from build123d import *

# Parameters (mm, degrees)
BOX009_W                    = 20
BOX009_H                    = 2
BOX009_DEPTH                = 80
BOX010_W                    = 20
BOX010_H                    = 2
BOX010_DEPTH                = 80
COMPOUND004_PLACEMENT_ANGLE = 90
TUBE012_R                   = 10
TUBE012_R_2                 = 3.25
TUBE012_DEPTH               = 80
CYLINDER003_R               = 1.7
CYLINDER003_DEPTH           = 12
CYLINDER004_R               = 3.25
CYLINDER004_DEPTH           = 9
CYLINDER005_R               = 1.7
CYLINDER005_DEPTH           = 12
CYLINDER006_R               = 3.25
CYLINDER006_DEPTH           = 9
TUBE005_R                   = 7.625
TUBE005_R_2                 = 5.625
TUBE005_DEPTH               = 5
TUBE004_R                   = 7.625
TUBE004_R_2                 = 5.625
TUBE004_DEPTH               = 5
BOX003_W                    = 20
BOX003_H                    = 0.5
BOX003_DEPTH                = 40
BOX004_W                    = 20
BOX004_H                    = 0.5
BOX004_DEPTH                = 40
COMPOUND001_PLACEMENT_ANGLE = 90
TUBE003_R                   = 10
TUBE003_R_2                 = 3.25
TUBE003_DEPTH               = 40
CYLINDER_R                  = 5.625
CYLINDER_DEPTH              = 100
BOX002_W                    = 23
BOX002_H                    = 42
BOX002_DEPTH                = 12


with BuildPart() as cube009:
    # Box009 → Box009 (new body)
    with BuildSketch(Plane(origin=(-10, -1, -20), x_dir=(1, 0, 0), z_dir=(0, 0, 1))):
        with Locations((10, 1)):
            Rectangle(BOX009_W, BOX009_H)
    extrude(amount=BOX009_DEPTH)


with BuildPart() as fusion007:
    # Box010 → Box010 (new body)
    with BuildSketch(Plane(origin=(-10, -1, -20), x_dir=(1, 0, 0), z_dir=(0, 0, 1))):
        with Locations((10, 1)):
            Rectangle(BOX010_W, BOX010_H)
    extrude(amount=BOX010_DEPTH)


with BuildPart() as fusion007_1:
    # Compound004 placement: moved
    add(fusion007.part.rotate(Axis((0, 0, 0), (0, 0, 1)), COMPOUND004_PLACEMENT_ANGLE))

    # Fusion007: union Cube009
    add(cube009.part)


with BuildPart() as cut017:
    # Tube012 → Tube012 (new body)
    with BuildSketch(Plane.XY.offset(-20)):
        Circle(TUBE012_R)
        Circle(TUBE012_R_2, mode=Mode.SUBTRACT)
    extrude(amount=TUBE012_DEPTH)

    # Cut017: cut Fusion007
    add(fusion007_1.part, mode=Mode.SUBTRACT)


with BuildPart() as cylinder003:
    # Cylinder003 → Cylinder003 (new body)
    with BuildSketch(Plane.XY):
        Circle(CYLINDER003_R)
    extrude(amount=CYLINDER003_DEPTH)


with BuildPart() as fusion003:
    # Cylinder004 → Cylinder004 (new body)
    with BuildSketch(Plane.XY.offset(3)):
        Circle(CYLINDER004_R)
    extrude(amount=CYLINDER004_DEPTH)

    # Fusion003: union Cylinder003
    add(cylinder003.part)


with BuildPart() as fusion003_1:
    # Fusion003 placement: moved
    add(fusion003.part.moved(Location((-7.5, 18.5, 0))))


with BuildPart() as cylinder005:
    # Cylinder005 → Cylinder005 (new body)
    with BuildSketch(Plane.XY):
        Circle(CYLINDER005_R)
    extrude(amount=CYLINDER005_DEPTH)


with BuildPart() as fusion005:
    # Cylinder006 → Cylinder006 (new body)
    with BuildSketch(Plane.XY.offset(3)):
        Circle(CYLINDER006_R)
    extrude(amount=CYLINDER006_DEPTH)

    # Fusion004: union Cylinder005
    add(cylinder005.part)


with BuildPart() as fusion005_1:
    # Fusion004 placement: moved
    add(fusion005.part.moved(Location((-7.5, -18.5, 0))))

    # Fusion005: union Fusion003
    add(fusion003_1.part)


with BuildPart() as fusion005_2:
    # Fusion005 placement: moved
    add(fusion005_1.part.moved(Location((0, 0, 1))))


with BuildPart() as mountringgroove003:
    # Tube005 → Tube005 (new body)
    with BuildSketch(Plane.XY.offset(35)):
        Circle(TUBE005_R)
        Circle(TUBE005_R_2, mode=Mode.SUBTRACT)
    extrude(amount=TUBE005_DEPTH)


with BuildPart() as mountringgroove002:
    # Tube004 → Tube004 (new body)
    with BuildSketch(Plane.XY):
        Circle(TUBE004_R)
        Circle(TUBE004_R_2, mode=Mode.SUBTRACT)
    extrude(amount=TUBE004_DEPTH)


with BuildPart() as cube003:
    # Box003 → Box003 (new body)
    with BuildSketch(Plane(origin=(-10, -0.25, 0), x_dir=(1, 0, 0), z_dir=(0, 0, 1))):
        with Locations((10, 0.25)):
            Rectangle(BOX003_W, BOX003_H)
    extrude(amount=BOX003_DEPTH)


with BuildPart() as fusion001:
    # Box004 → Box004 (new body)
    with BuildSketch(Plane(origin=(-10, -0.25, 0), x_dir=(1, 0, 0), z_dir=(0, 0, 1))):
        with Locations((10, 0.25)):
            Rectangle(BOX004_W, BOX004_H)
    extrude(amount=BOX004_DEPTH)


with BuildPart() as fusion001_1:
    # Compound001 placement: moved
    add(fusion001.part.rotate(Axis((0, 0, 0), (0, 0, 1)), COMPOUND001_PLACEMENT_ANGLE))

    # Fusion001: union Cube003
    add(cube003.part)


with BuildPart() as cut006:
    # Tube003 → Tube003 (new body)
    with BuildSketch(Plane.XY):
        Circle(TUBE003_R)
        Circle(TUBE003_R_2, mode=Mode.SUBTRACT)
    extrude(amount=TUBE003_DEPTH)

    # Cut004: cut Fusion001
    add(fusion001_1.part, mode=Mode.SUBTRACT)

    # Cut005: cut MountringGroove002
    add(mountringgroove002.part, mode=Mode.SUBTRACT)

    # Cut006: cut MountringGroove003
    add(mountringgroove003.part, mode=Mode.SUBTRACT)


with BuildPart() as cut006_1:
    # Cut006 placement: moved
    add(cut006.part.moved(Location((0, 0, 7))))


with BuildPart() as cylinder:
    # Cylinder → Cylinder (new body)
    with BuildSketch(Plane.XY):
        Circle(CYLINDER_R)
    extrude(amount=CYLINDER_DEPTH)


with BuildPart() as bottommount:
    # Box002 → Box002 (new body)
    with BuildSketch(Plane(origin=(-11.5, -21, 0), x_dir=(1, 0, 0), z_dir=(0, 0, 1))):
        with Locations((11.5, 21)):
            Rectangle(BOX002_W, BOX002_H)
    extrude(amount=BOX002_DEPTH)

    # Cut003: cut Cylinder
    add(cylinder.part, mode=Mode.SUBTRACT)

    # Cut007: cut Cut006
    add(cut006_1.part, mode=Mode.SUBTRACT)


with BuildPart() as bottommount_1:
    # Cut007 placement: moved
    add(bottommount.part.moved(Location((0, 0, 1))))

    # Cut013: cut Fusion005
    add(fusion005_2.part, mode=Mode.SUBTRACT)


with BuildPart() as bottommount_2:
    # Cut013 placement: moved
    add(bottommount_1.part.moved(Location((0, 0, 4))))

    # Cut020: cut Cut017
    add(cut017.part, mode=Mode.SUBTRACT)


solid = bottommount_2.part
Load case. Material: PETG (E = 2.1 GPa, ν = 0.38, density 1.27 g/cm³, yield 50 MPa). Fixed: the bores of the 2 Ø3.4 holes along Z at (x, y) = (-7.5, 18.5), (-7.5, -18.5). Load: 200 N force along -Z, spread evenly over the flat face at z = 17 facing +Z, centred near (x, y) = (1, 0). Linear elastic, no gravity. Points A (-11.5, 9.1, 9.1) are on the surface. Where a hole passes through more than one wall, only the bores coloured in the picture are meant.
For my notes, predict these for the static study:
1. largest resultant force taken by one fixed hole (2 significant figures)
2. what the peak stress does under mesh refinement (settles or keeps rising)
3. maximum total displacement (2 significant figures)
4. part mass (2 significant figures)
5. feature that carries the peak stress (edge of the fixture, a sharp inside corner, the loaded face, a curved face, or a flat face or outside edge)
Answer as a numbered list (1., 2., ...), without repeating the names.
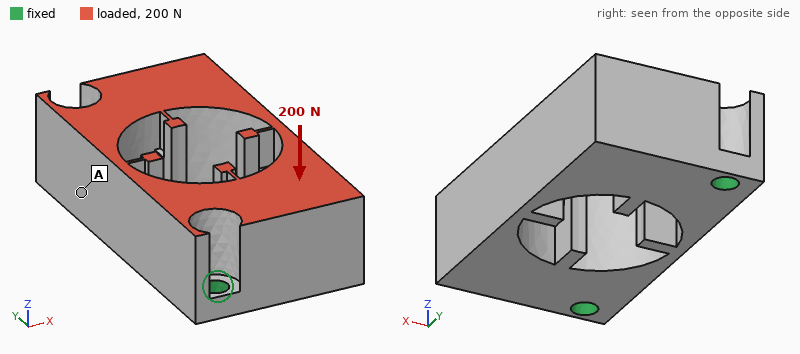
1. 110 N
2. keeps rising
3. 0.53 mm
4. 9.6 g
5. edge of the fixture
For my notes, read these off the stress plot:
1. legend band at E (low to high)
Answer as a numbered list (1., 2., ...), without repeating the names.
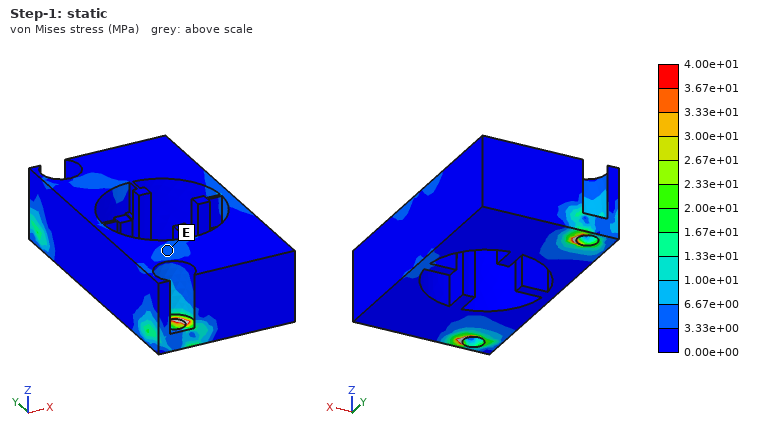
1. 3.33e+00 to 6.67e+00 MPa
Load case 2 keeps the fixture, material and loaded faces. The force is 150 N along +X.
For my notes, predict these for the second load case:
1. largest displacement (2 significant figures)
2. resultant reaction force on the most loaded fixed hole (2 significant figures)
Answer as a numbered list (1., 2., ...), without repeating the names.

1. 0.51 mm
2. 75 N
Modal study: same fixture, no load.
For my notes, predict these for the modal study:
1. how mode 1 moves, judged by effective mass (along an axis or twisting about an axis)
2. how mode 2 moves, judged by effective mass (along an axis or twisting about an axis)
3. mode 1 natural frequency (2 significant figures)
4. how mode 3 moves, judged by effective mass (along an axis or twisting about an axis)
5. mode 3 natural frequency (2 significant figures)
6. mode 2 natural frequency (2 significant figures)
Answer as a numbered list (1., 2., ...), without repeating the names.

1. along Z
2. along Y
3. 1100 Hz
4. twisting about X
5. 2900 Hz
6. 2500 Hz
